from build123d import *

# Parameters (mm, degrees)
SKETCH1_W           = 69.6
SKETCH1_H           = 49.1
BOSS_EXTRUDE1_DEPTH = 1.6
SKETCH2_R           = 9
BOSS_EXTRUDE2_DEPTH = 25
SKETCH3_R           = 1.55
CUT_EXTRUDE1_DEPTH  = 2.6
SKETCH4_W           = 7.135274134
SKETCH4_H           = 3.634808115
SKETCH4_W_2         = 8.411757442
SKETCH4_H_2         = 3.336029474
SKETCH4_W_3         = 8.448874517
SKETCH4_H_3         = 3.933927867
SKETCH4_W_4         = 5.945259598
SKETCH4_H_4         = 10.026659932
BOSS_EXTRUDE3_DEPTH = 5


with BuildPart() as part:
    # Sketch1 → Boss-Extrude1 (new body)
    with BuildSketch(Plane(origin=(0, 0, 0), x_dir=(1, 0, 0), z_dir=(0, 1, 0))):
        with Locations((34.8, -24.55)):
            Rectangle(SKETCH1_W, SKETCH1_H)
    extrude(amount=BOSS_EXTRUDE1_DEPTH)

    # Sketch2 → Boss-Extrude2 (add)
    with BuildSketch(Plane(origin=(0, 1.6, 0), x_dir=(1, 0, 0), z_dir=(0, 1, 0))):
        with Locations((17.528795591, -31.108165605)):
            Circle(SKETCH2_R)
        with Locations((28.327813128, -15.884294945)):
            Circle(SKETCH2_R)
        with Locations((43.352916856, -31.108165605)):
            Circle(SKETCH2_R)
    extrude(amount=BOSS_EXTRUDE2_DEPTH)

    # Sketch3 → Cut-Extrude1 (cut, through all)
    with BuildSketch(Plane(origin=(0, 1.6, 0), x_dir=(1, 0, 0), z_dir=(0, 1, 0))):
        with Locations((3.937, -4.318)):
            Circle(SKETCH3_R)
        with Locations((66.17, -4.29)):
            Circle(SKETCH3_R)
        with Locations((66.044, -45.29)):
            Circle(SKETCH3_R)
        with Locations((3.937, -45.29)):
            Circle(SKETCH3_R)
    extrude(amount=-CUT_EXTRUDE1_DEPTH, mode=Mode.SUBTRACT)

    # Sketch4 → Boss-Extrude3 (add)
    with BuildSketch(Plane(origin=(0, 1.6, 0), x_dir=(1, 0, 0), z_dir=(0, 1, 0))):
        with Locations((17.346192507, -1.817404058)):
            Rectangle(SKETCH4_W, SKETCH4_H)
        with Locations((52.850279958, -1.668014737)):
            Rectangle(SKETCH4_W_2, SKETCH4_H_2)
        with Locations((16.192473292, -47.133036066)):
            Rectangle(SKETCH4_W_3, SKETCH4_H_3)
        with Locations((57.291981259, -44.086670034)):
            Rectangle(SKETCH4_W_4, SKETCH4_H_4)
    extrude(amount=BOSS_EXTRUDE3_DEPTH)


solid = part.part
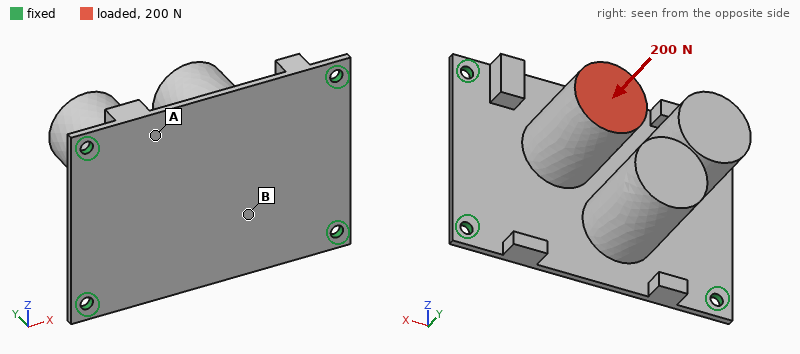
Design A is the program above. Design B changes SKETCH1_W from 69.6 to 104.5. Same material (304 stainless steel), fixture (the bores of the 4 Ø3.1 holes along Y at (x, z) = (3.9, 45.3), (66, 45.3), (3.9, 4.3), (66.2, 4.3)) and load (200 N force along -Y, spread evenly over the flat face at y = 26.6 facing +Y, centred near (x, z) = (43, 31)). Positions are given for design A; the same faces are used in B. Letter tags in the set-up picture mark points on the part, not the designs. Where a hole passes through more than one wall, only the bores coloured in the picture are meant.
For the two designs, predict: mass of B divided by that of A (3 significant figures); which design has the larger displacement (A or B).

1.11
A
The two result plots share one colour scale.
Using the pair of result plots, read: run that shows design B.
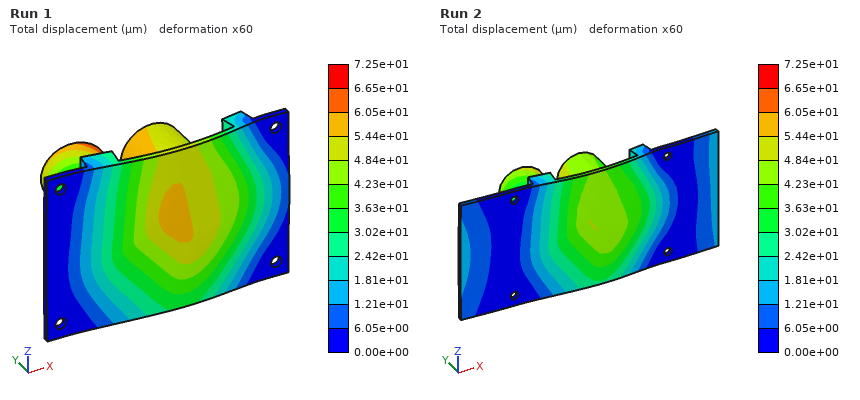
Run 2
